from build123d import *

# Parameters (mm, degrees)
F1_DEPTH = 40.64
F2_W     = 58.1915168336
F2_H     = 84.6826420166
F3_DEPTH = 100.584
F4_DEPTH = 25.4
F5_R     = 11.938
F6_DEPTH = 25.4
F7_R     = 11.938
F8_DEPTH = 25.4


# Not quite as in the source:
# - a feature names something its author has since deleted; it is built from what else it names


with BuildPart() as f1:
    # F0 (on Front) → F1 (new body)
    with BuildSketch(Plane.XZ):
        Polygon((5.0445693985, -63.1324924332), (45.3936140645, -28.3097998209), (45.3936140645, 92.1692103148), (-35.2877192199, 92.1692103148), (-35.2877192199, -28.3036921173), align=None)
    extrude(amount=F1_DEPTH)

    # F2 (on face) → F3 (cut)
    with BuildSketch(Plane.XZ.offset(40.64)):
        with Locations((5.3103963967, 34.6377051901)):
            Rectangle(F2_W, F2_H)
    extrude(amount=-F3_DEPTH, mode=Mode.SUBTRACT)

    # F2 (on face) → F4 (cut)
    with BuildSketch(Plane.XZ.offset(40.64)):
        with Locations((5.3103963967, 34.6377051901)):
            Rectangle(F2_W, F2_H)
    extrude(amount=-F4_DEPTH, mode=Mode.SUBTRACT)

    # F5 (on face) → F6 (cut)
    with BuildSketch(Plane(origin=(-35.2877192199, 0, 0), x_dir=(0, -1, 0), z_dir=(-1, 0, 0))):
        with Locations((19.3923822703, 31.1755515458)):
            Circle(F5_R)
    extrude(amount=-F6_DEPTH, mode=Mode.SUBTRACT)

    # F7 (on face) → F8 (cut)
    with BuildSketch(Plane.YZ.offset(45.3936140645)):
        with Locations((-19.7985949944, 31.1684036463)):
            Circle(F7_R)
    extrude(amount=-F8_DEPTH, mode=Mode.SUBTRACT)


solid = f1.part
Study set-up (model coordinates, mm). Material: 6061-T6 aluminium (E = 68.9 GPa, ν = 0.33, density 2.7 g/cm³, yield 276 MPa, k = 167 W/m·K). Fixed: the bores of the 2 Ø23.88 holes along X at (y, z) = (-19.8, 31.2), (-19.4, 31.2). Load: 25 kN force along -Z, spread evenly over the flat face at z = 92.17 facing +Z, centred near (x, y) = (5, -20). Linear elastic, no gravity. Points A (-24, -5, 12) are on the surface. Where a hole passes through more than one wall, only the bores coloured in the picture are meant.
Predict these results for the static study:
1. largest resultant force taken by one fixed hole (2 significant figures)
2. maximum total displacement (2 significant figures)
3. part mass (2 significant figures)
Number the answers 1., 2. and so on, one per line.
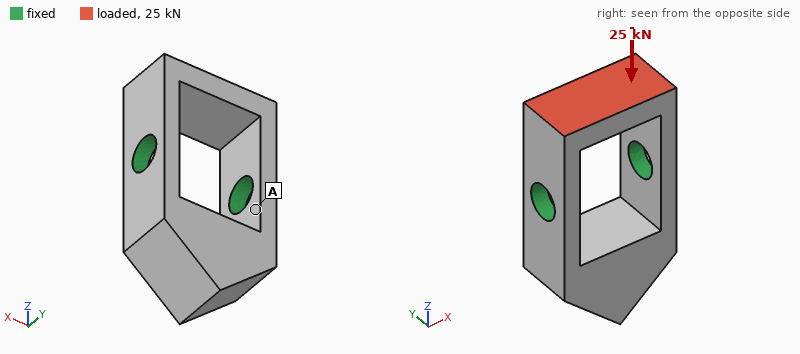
1. 13 kN
2. 82 µm
3. 650 g
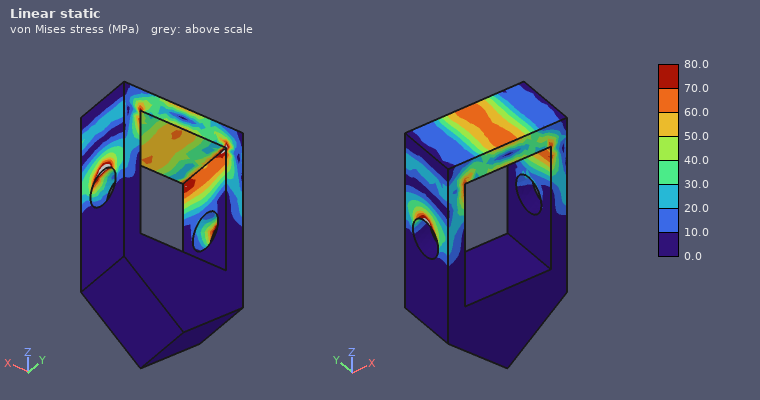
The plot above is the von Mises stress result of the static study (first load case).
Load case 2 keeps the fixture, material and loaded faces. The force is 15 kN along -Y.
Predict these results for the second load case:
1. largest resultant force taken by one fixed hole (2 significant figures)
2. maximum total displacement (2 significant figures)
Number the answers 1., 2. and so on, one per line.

1. 7.6 kN
2. 0.19 mm
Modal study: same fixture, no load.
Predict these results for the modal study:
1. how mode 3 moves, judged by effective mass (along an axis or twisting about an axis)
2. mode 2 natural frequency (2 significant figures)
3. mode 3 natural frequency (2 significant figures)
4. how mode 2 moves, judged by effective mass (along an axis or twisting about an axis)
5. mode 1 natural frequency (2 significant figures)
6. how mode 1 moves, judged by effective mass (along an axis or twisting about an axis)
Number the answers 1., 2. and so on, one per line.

1. along X
2. 3100 Hz
3. 3500 Hz
4. along X
5. 2600 Hz
6. along Y
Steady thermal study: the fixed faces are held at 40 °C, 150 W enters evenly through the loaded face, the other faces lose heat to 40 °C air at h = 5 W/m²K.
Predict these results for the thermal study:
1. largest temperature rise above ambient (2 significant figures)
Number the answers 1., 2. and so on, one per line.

1. 51 K
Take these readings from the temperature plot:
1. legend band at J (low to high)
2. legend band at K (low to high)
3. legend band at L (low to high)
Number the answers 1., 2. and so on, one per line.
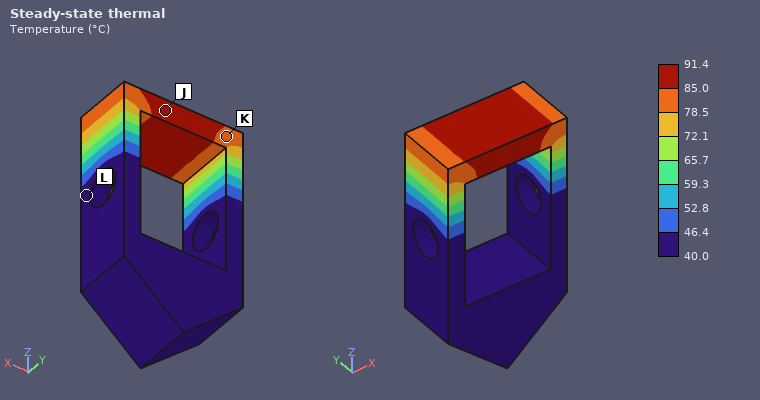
1. 85.0 to 91.4 °C
2. 78.5 to 85.0 °C
3. 40.0 to 46.4 °C
